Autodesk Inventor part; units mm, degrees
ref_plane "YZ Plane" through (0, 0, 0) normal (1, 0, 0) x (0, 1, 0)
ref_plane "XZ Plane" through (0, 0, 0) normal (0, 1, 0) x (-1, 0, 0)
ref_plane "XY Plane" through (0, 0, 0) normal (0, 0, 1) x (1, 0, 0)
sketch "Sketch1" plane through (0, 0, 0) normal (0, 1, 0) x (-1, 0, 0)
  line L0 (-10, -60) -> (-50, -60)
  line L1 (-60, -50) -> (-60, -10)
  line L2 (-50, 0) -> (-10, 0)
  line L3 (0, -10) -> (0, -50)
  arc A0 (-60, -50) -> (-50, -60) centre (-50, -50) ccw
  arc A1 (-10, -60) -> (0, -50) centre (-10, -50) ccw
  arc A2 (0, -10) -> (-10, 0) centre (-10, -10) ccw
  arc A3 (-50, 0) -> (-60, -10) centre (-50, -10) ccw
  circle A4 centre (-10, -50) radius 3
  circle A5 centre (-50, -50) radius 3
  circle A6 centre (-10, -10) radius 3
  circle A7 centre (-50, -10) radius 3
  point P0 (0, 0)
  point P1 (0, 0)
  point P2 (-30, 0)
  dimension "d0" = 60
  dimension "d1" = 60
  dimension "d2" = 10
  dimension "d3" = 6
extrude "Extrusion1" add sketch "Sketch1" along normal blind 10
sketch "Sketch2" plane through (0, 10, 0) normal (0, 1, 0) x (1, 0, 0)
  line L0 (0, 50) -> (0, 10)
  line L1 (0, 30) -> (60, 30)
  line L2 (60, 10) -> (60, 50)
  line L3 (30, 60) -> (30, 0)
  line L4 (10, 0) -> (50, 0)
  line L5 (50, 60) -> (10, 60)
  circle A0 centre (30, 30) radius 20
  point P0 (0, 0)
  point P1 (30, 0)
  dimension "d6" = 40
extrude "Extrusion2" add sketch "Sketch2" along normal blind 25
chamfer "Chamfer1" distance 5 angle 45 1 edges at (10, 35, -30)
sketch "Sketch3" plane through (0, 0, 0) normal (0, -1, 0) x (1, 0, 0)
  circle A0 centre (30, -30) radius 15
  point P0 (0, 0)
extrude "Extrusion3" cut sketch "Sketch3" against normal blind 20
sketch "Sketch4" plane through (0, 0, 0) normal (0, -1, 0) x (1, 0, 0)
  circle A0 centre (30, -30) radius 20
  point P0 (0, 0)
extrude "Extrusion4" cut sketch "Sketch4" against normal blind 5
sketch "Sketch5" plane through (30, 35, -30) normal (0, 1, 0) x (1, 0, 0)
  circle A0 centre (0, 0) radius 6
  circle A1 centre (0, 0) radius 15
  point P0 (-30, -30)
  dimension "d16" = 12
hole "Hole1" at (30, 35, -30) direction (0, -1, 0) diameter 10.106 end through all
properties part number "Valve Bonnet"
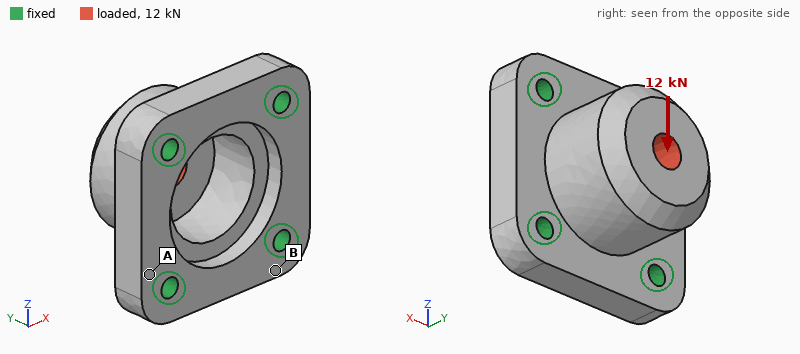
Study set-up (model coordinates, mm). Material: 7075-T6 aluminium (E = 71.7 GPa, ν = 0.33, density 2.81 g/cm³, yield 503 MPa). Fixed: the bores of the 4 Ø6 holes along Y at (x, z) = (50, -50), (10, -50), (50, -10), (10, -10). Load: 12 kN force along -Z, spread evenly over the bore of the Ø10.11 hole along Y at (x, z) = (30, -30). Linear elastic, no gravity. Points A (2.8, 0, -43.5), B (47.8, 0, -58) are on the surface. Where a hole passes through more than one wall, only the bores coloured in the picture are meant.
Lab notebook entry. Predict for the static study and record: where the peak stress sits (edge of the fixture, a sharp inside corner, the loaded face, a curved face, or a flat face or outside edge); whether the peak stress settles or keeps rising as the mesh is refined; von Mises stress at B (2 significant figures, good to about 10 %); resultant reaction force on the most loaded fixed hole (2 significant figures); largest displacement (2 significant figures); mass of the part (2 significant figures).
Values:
edge of the fixture
keeps rising
22 MPa
4.7 kN
56 µm
130 g
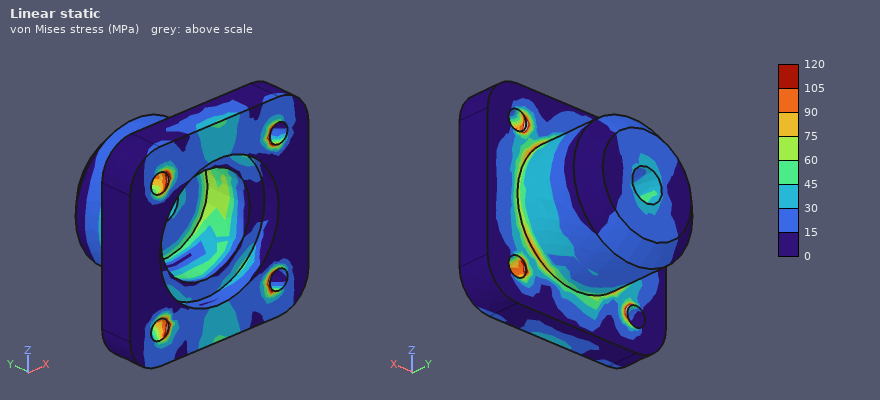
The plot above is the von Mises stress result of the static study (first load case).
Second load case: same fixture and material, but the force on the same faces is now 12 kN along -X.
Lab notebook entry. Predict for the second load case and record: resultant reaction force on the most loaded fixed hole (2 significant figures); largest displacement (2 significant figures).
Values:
4.7 kN
56 µm
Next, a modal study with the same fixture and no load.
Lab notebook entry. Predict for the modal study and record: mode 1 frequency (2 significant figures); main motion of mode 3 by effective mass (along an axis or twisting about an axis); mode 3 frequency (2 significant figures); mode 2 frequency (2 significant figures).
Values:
12 kHz
along Y
16 kHz
12 kHz
